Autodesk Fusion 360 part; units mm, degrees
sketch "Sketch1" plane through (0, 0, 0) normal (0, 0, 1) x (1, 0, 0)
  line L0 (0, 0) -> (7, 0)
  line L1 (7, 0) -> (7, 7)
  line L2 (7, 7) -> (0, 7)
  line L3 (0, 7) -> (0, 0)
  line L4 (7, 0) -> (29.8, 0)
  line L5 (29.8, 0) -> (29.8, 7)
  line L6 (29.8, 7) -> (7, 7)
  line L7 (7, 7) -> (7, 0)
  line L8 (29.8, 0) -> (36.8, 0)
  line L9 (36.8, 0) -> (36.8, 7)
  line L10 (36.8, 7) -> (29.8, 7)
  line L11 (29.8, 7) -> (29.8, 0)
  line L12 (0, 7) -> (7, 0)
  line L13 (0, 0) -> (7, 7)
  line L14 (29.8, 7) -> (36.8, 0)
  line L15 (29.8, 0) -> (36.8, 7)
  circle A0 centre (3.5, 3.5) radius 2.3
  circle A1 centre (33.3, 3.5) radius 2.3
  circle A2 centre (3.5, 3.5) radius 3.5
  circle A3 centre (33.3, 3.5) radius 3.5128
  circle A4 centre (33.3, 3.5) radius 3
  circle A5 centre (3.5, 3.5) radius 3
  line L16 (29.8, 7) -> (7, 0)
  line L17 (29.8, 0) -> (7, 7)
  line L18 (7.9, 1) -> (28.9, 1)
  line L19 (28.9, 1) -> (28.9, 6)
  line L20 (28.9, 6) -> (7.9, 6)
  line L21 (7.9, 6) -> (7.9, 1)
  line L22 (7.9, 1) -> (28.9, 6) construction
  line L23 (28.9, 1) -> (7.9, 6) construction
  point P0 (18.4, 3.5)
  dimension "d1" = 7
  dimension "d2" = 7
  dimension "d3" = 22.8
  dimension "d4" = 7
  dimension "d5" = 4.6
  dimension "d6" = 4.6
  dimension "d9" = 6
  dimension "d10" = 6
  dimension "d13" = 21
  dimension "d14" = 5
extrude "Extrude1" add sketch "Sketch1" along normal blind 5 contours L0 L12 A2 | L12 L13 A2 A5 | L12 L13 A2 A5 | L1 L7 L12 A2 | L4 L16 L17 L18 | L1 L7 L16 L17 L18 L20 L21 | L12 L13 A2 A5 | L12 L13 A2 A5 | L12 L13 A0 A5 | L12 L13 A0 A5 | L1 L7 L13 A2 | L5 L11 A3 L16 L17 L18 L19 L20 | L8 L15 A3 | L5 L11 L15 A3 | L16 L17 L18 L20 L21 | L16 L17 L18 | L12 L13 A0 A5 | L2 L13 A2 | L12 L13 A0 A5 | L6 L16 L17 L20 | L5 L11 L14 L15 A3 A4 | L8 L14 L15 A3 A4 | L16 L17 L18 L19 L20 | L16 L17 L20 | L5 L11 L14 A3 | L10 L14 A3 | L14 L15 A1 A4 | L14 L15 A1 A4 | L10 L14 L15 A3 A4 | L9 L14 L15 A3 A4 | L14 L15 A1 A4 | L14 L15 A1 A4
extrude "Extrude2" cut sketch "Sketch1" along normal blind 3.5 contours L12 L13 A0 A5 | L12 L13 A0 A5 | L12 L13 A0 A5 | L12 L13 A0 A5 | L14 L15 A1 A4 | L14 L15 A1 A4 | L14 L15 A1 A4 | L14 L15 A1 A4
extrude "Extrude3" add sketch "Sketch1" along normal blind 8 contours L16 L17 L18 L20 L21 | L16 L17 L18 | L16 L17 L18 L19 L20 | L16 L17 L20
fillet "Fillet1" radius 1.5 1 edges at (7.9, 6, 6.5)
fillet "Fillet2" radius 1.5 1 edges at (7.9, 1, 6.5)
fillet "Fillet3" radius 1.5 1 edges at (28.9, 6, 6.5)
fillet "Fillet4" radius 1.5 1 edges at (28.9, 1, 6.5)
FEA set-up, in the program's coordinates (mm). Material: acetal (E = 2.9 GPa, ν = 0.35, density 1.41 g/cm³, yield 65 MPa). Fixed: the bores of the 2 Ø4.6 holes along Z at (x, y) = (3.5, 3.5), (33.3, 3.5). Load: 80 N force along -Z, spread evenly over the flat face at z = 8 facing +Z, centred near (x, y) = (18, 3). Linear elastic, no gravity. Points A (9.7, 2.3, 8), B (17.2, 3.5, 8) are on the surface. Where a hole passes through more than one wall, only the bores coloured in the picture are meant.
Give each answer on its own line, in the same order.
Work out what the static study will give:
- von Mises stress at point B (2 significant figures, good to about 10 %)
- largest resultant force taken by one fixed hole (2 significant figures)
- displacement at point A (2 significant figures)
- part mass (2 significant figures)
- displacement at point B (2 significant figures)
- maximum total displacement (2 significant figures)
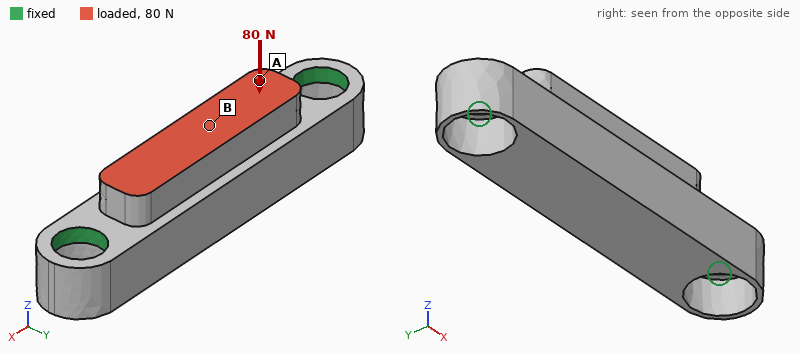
3.8 MPa
42 N
23 µm
1.8 g
35 µm
36 µm
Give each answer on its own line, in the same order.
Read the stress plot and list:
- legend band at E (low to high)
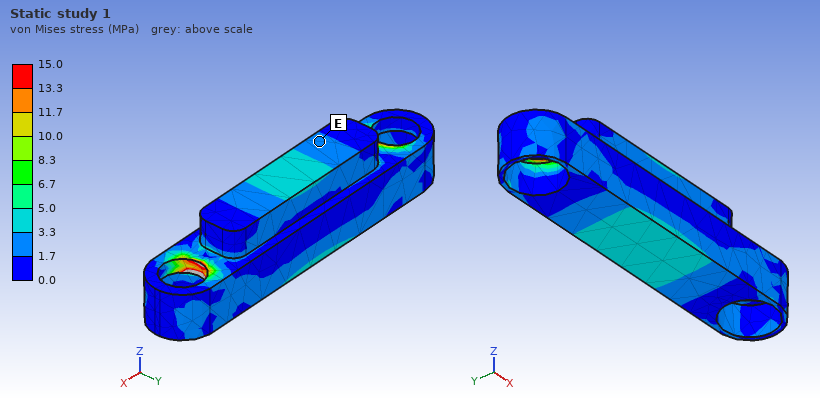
1.7 to 3.3 MPa
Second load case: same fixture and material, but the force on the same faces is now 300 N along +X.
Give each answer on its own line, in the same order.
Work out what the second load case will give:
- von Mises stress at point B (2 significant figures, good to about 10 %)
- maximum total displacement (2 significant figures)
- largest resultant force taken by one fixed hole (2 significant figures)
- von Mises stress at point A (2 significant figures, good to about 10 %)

5.1 MPa
50 µm
160 N
6.2 MPa
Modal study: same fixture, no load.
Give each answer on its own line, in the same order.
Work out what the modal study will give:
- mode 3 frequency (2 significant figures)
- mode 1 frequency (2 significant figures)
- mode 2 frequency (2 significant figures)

7700 Hz
6700 Hz
6800 Hz
